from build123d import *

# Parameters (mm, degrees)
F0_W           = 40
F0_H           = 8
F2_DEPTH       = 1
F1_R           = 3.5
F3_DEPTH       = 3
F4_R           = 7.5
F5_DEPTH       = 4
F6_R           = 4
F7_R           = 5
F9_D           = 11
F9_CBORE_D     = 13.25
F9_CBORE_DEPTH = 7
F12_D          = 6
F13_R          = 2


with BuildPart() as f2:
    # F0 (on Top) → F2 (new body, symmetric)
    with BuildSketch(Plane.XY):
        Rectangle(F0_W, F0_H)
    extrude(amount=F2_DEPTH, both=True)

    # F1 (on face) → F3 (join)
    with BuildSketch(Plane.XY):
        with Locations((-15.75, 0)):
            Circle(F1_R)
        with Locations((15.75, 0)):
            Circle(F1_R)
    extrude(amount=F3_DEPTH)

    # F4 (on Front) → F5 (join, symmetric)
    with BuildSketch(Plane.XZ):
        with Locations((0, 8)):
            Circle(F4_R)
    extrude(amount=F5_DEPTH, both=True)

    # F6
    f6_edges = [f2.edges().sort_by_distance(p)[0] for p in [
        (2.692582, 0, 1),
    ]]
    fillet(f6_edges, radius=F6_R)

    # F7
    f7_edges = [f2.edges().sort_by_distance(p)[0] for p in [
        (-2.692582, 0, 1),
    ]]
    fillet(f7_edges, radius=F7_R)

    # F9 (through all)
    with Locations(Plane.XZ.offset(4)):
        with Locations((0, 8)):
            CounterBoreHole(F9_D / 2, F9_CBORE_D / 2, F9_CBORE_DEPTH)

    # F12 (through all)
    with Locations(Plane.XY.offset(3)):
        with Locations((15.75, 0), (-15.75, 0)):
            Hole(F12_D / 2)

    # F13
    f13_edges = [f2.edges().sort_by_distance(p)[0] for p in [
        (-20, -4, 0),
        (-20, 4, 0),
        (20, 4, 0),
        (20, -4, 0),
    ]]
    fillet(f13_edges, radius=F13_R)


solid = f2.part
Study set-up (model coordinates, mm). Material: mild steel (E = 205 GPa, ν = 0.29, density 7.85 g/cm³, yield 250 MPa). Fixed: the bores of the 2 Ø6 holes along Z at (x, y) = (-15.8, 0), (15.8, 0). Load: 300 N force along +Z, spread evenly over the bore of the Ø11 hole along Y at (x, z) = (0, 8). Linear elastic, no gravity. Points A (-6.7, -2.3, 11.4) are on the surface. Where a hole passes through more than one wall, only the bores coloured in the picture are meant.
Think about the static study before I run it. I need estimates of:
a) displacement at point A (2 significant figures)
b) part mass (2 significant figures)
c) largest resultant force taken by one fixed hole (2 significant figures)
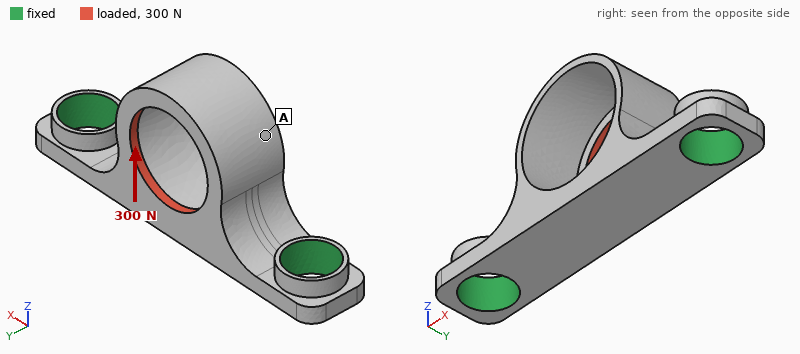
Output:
11 µm
8.6 g
190 N
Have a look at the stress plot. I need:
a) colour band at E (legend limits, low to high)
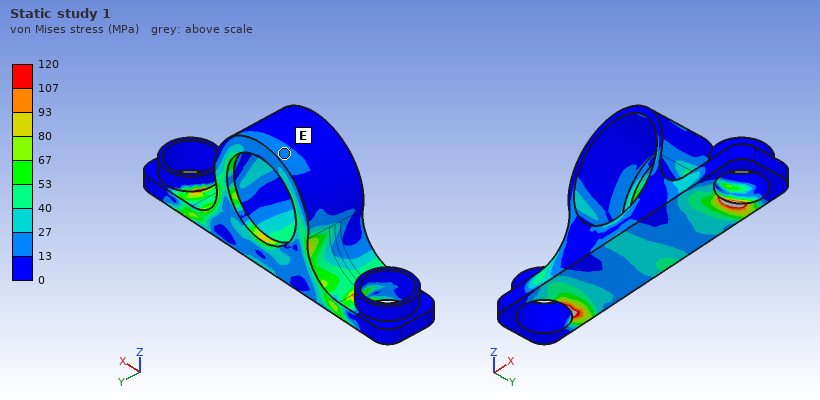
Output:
13 to 27 MPa
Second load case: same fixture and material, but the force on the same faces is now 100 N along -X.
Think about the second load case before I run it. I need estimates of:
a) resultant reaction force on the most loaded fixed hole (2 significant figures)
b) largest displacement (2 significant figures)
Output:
64 N
6.5 µm
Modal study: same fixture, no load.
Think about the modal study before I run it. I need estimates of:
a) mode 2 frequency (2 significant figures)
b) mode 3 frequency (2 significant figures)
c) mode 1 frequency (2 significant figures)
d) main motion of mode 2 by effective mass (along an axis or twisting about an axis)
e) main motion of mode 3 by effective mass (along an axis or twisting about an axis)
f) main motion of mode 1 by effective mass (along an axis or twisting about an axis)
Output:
12 kHz
15 kHz
9300 Hz
along X
along Z
along Y
